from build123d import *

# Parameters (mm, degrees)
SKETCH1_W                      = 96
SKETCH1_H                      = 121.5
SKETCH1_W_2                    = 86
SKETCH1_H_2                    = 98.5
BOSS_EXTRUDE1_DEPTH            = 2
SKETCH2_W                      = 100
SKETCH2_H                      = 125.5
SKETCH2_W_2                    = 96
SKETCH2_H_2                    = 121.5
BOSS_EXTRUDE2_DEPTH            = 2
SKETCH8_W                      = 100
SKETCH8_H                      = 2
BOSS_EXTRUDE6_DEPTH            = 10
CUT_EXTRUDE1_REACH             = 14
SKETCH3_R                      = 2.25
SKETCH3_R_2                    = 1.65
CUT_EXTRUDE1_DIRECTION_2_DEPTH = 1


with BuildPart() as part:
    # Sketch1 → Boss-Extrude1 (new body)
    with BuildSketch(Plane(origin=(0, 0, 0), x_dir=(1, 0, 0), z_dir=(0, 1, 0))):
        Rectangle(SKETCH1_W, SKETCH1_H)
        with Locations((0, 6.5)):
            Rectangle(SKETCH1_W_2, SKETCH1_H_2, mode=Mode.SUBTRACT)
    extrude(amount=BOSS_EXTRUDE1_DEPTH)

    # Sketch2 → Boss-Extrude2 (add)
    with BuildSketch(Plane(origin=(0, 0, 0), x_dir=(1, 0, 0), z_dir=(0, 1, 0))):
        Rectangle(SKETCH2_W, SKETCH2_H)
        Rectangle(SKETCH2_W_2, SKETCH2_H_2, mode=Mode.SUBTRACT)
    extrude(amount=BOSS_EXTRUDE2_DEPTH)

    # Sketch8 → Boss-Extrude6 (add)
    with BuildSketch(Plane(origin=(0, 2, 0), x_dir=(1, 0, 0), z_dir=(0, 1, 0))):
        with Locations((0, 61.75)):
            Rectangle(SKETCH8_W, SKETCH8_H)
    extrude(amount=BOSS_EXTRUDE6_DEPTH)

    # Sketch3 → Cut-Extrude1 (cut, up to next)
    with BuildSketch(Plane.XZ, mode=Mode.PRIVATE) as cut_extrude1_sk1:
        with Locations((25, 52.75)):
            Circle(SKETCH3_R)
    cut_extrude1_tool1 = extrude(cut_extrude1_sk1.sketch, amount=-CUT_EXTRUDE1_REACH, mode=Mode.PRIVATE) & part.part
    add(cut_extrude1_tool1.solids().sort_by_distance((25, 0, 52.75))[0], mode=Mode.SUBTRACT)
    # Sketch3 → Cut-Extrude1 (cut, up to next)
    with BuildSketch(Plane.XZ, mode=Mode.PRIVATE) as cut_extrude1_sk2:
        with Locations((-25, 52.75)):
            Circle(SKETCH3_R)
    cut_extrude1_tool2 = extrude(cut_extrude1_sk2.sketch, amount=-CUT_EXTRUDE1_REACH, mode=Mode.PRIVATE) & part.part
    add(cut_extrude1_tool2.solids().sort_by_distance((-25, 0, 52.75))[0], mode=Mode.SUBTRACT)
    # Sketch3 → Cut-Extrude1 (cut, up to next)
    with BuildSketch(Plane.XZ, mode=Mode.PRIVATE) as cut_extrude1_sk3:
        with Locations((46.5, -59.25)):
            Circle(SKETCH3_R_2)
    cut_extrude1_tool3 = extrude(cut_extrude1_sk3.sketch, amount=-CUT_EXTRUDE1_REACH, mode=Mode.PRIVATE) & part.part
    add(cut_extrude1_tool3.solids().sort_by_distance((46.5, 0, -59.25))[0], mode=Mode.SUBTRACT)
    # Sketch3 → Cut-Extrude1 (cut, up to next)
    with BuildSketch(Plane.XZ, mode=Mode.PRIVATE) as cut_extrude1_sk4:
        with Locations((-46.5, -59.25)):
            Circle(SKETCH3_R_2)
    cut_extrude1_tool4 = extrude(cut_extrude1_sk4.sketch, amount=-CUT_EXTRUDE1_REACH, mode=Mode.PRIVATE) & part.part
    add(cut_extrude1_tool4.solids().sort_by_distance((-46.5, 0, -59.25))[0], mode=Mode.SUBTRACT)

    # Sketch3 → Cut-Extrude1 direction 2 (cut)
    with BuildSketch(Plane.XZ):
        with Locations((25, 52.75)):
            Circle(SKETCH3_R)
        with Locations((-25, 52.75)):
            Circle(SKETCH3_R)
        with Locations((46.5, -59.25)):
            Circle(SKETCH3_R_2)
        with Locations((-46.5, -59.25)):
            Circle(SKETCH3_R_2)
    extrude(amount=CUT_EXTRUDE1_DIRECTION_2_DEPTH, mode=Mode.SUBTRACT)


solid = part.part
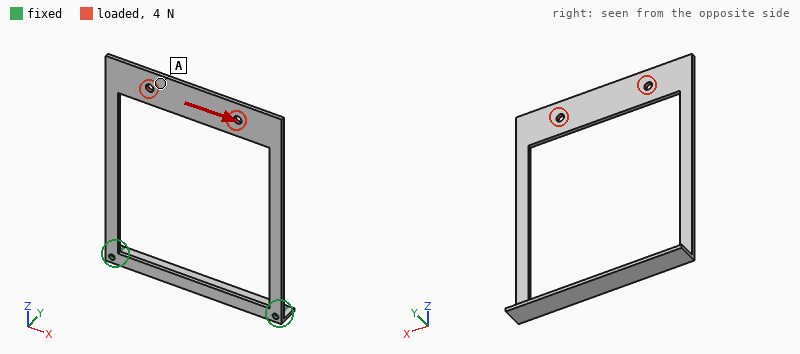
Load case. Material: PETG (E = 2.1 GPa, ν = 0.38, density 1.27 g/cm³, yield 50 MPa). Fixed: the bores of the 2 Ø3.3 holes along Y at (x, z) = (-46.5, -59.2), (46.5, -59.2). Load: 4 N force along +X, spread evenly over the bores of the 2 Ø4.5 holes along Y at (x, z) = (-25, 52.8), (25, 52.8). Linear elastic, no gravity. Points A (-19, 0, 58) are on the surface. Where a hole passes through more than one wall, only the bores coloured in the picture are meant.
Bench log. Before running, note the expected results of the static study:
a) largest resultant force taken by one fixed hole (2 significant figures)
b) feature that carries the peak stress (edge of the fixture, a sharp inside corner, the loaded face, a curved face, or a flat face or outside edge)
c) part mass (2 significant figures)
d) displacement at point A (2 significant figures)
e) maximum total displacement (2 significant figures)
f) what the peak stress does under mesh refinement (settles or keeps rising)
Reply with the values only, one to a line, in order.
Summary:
3.5 N
edge of the fixture
13 g
1.7 mm
1.7 mm
keeps rising
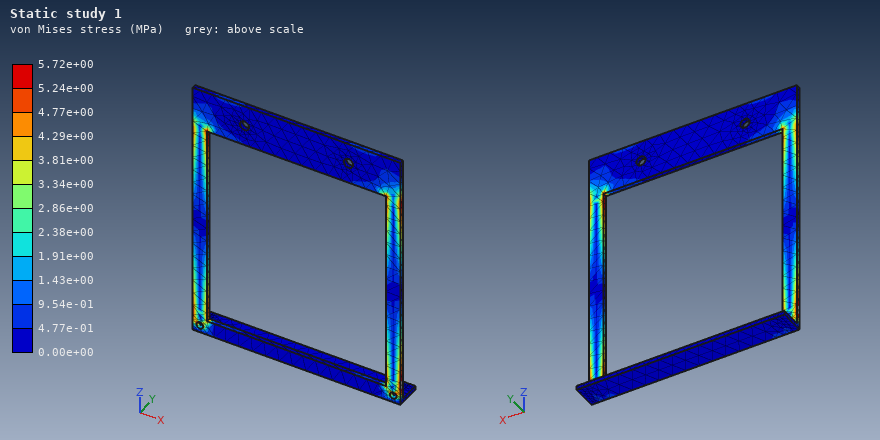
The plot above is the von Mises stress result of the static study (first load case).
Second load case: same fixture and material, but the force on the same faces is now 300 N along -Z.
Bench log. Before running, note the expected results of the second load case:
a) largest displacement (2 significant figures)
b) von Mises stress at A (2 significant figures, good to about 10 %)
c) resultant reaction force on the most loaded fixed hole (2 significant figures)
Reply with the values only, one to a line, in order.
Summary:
1.8 mm
10 MPa
150 N
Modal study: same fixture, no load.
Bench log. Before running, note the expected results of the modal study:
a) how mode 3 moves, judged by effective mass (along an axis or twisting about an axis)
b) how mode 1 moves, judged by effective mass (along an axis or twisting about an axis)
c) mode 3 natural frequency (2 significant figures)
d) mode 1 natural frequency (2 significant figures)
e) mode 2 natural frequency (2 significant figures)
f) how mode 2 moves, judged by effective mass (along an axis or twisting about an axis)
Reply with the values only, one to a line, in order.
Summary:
along X
along Y
98 Hz
14 Hz
46 Hz
twisting about Z
